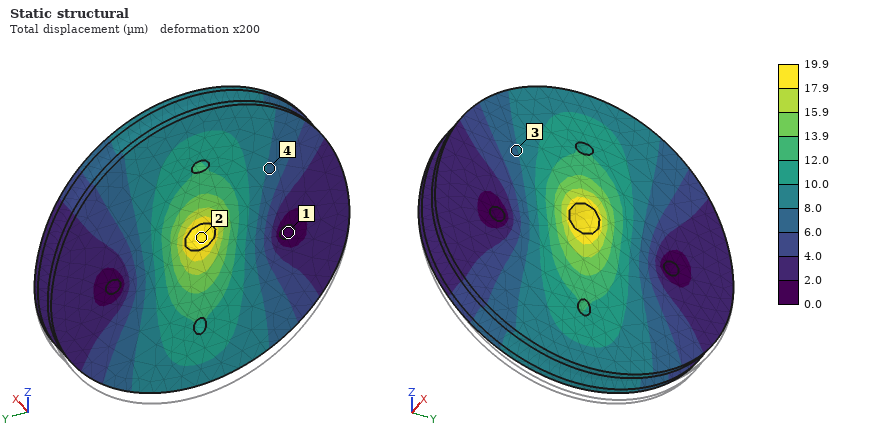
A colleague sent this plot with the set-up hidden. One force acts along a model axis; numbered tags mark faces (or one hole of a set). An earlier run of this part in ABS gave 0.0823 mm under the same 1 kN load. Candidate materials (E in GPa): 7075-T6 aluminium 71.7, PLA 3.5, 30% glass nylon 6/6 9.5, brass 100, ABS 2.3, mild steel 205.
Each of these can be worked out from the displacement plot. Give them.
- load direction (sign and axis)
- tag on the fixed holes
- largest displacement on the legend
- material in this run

+Z
1
19.9 µm
30% glass nylon 6/6
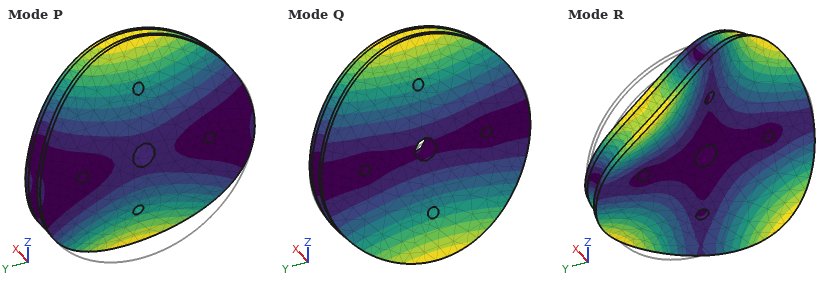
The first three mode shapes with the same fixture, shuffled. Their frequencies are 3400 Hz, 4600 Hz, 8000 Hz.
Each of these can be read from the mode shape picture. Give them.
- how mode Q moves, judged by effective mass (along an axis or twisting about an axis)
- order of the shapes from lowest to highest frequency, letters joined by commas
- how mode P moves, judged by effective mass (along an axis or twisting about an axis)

twisting about Y
Q, P, R
along X
